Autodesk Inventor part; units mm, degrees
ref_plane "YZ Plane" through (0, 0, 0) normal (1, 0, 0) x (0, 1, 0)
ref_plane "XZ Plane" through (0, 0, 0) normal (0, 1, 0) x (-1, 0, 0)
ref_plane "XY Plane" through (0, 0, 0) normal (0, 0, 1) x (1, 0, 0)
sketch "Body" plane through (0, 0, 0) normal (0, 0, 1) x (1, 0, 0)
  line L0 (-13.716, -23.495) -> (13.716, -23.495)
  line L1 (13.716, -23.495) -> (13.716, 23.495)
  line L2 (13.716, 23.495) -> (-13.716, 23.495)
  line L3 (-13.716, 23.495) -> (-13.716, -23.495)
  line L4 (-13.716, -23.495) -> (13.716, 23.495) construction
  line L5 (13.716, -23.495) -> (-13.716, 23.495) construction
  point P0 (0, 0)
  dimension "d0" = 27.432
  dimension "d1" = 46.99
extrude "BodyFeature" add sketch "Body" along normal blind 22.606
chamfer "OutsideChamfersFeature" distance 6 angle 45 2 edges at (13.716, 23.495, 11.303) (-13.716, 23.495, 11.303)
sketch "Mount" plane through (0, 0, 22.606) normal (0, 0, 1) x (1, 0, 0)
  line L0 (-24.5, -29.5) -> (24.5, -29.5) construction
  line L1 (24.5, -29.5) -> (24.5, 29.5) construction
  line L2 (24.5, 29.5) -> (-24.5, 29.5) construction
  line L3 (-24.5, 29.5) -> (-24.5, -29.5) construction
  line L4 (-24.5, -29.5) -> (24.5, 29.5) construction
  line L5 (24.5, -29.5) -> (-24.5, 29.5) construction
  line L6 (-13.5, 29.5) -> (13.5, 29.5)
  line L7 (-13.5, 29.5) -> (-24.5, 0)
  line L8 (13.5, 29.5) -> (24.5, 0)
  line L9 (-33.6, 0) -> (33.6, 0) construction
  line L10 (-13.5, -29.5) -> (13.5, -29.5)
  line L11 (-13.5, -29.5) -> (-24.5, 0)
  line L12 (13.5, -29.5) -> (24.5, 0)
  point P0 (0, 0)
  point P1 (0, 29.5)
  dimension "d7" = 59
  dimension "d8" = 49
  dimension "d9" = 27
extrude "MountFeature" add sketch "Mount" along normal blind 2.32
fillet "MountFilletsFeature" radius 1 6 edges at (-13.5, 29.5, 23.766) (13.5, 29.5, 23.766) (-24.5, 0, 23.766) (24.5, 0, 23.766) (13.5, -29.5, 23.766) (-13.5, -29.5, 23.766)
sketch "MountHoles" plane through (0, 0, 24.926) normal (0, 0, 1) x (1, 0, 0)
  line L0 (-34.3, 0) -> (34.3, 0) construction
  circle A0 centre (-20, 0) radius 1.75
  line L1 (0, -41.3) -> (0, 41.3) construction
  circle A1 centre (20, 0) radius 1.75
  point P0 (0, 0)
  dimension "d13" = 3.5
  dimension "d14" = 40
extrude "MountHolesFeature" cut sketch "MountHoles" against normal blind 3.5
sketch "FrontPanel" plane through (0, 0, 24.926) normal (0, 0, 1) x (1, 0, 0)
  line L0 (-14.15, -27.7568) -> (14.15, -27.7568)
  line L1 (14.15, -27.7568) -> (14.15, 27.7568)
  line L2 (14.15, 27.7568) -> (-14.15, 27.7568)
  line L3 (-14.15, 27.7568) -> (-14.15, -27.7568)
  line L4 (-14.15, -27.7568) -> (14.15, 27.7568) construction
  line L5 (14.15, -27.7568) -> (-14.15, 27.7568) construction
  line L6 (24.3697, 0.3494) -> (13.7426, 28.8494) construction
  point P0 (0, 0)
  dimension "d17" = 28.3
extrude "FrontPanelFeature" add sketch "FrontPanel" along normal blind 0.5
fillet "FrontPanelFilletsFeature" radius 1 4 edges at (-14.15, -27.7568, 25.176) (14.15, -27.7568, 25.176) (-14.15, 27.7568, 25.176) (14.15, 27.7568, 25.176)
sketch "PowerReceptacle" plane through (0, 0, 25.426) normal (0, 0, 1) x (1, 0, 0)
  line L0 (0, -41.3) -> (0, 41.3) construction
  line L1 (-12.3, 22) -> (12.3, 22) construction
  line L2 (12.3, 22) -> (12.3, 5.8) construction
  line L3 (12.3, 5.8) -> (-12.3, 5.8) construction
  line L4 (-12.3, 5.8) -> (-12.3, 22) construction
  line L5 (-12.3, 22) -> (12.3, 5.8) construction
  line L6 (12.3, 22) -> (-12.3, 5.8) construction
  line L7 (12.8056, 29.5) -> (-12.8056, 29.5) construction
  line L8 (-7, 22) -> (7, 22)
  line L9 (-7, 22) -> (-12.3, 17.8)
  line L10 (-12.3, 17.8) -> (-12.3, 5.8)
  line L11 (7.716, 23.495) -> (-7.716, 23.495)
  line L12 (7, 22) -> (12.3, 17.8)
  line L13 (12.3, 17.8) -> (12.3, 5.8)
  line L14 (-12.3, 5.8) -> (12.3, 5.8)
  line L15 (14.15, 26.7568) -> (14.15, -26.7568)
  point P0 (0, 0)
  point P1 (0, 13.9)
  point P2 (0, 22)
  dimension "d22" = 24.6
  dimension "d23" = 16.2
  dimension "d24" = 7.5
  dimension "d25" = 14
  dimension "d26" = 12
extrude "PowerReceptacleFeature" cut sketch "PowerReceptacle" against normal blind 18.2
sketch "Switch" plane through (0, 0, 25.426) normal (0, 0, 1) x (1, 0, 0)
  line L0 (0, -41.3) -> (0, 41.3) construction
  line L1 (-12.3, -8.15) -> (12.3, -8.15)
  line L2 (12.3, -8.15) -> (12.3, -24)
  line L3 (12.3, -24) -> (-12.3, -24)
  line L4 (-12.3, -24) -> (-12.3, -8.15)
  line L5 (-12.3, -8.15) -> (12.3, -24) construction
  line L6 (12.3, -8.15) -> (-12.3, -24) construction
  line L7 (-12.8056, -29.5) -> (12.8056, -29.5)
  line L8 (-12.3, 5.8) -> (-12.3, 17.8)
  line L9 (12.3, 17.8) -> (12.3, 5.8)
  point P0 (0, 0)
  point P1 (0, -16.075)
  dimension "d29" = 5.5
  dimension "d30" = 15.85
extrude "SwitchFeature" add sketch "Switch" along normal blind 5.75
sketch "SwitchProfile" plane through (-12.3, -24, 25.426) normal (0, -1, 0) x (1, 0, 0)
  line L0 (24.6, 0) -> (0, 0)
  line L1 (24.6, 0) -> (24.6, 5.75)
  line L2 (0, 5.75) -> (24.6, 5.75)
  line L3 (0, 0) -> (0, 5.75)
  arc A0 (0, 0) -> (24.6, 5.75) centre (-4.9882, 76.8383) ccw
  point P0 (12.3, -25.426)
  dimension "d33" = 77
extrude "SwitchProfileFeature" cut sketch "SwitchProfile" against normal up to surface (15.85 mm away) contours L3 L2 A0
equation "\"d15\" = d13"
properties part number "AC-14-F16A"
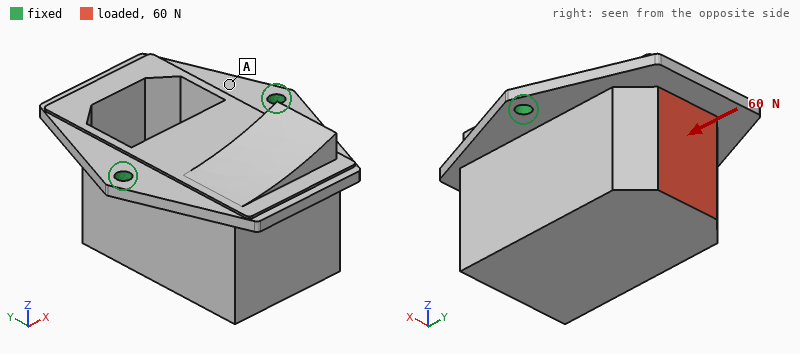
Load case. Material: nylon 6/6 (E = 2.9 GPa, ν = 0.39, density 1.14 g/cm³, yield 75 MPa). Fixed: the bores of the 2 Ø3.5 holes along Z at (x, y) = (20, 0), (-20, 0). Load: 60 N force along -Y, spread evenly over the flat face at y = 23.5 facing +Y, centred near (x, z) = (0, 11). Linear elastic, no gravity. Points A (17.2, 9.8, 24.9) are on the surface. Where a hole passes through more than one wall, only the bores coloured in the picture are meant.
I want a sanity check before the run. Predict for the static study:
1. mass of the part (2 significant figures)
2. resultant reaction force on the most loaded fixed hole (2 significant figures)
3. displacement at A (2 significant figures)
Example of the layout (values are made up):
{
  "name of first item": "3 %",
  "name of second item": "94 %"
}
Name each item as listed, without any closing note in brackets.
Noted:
{
  "mass of the part": "32 g",
  "resultant reaction force on the most loaded fixed hole": "30 N",
  "displacement at A": "0.16 mm"
}
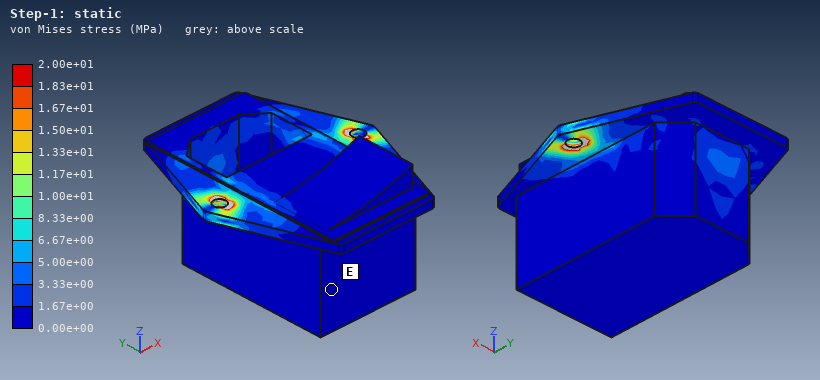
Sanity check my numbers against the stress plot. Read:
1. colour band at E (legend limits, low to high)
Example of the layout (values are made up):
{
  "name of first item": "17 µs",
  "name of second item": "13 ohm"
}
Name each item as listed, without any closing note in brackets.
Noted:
{
  "colour band at E": "0.00e+00 to 1.67e+00 MPa"
}
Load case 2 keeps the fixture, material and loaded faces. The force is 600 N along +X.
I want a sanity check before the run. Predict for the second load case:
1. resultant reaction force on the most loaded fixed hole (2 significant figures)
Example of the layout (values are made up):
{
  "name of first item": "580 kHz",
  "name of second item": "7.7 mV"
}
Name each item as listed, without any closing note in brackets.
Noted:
{
  "resultant reaction force on the most loaded fixed hole": "510 N"
}
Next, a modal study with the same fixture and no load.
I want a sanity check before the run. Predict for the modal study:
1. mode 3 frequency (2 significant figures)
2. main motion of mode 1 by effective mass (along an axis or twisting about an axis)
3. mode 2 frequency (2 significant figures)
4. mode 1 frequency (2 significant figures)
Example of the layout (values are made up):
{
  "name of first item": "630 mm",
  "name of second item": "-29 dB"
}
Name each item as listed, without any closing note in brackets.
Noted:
{
  "mode 3 frequency": "1500 Hz",
  "main motion of mode 1 by effective mass": "along Y",
  "mode 2 frequency": "1400 Hz",
  "mode 1 frequency": "290 Hz"
}
